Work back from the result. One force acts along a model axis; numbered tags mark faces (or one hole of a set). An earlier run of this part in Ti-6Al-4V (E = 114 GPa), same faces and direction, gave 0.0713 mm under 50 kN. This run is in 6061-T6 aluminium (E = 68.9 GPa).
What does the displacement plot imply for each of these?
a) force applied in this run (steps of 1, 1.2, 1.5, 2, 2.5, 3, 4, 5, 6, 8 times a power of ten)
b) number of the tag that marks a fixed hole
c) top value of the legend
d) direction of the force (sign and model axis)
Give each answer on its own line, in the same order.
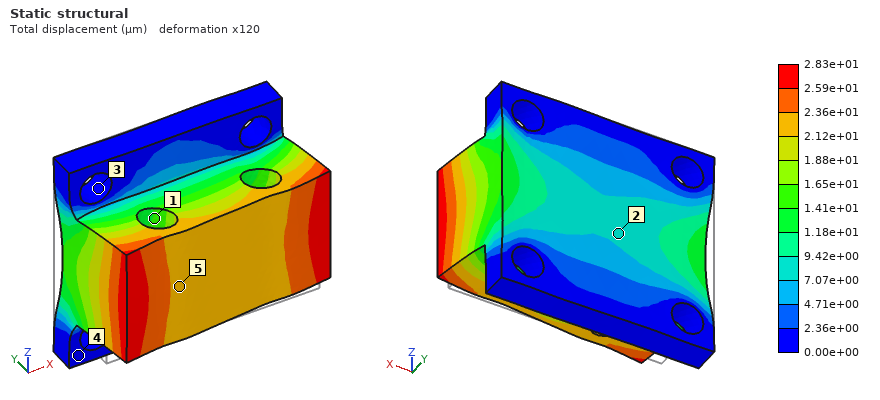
12 kN
3
2.83e+01 µm
+X
